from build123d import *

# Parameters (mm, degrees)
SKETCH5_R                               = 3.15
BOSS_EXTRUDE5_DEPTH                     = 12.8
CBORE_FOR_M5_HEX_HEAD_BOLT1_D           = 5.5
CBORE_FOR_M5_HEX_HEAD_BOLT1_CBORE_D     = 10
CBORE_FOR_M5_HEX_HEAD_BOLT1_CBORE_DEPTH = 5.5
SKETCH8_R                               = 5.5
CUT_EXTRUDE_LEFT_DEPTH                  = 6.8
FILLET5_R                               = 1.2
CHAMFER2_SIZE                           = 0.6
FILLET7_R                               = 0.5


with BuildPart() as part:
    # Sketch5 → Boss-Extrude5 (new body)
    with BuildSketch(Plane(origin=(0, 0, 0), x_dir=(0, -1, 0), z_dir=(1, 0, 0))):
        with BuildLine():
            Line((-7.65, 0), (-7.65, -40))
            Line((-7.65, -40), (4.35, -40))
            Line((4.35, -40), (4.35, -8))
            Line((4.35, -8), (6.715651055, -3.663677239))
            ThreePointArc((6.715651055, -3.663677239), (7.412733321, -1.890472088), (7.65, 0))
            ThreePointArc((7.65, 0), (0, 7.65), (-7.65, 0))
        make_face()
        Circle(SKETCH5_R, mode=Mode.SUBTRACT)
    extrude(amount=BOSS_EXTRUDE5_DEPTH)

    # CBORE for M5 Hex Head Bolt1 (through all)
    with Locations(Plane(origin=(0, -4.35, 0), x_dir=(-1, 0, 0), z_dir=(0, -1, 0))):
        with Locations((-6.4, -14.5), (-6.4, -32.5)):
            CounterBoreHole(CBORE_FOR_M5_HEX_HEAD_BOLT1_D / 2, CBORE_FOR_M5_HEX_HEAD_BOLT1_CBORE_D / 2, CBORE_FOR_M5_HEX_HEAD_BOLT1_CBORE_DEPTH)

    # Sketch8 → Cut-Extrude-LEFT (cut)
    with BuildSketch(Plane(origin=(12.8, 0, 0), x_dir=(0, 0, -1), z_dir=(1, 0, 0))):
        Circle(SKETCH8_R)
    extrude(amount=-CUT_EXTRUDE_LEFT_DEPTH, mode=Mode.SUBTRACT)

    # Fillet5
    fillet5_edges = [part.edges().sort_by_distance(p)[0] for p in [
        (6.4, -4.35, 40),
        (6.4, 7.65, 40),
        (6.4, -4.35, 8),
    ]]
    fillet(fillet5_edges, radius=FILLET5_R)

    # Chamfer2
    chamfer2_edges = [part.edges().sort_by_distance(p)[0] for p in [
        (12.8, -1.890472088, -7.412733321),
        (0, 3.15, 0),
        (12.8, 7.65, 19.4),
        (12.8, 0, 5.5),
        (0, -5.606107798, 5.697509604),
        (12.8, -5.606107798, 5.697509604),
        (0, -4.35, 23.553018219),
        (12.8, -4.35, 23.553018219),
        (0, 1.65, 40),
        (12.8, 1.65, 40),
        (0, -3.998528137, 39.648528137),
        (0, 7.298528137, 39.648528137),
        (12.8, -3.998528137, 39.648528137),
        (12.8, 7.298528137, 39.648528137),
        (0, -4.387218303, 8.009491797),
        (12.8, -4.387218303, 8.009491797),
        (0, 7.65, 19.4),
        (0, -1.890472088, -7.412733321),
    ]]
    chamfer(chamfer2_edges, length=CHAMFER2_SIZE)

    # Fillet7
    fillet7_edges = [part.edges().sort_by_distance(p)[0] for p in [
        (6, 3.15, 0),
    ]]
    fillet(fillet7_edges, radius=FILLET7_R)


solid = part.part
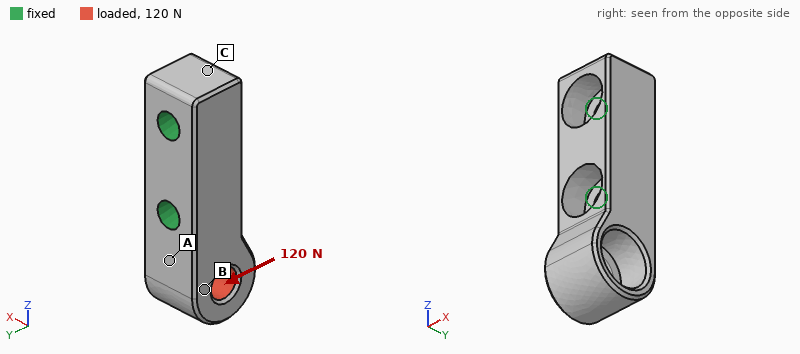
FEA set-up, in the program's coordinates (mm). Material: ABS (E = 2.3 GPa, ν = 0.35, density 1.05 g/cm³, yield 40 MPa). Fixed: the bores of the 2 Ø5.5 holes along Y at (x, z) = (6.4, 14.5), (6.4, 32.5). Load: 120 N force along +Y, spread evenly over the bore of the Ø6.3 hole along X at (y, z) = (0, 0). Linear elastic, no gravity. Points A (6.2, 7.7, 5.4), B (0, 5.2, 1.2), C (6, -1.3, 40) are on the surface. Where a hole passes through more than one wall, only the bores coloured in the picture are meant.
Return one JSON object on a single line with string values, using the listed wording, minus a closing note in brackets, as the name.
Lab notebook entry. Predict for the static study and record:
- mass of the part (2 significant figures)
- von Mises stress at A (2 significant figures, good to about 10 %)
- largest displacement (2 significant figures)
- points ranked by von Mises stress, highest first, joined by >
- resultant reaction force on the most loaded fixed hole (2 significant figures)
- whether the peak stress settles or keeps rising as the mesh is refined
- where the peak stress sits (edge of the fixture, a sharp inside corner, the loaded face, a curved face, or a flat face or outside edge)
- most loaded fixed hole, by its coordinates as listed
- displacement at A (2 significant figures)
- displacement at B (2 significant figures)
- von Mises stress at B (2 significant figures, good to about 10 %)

{"mass of the part": "5.7 g", "von Mises stress at A": "5.0 MPa", "largest displacement": "0.17 mm", "points ranked by von Mises stress, highest first, joined by >": "A > B > C", "resultant reaction force on the most loaded fixed hole": "160 N", "whether the peak stress settles or keeps rising as the mesh is refined": "keeps rising", "where the peak stress sits": "edge of the fixture", "most loaded fixed hole, by its coordinates as listed": "(6.4, 14.5)", "displacement at A": "0.051 mm", "displacement at B": "0.097 mm", "von Mises stress at B": "3.1 MPa"}
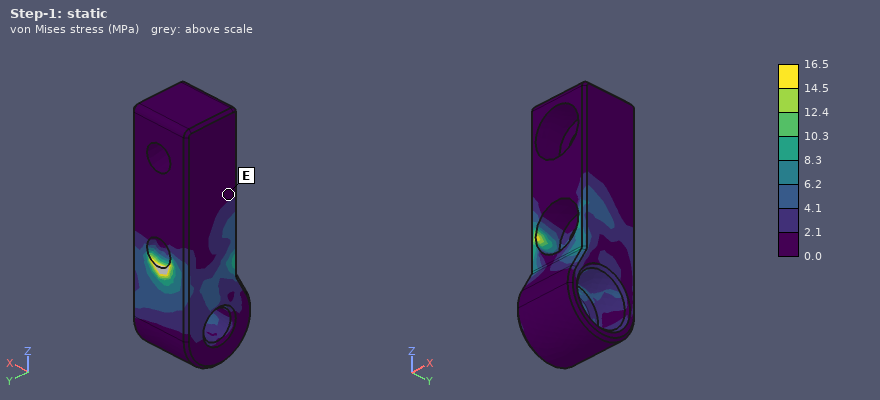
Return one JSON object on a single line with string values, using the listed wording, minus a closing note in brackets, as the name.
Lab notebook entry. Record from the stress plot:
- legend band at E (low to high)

{"legend band at E": "0.0 to 2.1 MPa"}
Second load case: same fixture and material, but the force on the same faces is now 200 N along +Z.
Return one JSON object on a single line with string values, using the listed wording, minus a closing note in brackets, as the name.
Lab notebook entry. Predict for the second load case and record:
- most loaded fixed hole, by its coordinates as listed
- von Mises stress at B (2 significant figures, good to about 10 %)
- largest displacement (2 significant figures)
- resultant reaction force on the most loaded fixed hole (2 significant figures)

{"most loaded fixed hole, by its coordinates as listed": "(6.4, 14.5)", "von Mises stress at B": "2.5 MPa", "largest displacement": "0.10 mm", "resultant reaction force on the most loaded fixed hole": "160 N"}
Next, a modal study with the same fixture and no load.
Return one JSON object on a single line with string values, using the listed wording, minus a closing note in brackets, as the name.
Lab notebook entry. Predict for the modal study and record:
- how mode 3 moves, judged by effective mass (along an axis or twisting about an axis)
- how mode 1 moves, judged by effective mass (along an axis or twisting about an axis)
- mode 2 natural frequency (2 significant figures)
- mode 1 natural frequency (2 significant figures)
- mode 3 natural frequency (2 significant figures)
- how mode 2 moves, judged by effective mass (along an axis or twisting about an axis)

{"how mode 3 moves, judged by effective mass": "twisting about Z", "how mode 1 moves, judged by effective mass": "along Y", "mode 2 natural frequency": "4400 Hz", "mode 1 natural frequency": "3700 Hz", "mode 3 natural frequency": "7500 Hz", "how mode 2 moves, judged by effective mass": "along X"}
